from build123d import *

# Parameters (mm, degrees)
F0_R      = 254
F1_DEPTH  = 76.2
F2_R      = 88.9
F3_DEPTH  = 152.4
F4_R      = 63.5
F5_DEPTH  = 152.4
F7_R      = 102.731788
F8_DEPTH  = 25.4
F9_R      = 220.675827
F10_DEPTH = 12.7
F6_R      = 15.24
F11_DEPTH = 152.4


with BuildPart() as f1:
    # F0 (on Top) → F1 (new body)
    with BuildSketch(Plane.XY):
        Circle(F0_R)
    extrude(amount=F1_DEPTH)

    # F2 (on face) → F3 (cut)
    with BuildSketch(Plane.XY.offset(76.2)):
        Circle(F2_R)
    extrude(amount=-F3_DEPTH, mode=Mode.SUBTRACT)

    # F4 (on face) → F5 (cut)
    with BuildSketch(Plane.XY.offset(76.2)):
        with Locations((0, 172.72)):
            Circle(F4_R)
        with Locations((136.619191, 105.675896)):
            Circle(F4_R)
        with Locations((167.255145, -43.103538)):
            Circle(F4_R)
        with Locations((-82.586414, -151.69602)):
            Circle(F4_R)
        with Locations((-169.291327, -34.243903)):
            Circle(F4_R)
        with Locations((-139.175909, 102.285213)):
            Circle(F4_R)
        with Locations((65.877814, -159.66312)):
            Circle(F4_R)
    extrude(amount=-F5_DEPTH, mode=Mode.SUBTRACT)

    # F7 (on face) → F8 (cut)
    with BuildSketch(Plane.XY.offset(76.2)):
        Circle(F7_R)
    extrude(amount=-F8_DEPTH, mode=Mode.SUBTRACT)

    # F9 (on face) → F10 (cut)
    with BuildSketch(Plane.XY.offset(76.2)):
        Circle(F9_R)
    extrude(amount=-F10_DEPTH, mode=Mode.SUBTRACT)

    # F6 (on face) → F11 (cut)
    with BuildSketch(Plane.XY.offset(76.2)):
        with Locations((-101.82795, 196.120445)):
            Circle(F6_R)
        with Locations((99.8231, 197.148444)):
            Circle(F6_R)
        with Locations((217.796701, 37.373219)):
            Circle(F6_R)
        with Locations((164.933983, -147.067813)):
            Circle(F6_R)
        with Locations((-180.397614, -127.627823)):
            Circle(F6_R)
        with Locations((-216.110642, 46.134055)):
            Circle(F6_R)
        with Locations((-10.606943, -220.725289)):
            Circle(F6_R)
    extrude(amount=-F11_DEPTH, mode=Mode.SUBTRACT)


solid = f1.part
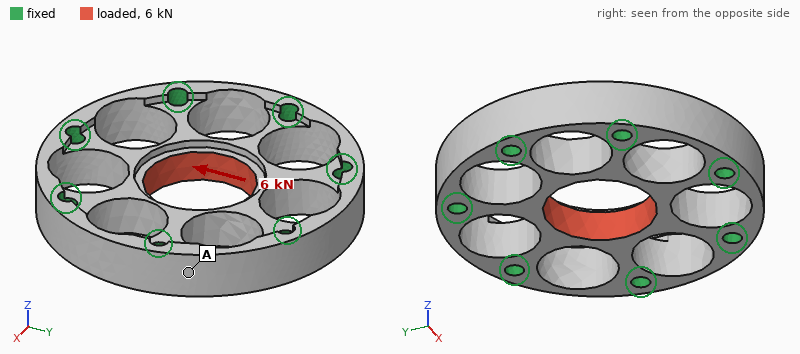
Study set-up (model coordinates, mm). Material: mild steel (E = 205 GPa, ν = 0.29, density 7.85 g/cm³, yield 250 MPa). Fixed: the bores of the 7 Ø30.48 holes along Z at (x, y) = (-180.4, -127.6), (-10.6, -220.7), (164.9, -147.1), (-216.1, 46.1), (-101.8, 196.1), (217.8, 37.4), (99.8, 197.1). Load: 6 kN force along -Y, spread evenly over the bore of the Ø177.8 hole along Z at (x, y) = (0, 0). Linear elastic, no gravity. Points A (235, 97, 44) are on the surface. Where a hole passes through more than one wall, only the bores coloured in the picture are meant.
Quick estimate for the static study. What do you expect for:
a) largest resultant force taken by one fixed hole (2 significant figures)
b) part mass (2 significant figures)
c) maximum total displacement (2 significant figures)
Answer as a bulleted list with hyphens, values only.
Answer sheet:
- 1.5 kN
- 45 kg
- 0.63 µm
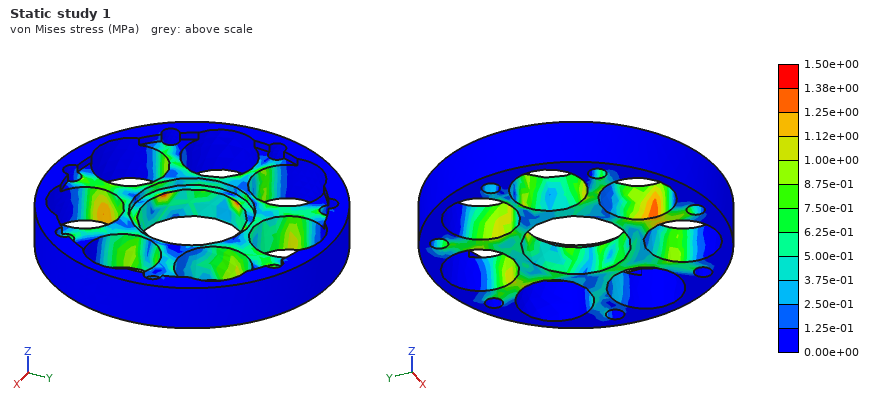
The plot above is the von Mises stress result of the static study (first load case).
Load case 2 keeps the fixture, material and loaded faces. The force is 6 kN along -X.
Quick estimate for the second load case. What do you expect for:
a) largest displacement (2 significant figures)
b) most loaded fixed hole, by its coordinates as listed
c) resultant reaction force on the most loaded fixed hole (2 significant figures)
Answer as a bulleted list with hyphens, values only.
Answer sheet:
- 0.67 µm
- (217.8, 37.4)
- 1.5 kN
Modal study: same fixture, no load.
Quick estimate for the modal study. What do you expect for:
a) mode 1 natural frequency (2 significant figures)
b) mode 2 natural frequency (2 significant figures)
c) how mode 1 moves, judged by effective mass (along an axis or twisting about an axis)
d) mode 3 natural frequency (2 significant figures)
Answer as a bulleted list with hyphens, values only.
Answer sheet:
- 2600 Hz
- 3300 Hz
- along Z
- 3400 Hz
